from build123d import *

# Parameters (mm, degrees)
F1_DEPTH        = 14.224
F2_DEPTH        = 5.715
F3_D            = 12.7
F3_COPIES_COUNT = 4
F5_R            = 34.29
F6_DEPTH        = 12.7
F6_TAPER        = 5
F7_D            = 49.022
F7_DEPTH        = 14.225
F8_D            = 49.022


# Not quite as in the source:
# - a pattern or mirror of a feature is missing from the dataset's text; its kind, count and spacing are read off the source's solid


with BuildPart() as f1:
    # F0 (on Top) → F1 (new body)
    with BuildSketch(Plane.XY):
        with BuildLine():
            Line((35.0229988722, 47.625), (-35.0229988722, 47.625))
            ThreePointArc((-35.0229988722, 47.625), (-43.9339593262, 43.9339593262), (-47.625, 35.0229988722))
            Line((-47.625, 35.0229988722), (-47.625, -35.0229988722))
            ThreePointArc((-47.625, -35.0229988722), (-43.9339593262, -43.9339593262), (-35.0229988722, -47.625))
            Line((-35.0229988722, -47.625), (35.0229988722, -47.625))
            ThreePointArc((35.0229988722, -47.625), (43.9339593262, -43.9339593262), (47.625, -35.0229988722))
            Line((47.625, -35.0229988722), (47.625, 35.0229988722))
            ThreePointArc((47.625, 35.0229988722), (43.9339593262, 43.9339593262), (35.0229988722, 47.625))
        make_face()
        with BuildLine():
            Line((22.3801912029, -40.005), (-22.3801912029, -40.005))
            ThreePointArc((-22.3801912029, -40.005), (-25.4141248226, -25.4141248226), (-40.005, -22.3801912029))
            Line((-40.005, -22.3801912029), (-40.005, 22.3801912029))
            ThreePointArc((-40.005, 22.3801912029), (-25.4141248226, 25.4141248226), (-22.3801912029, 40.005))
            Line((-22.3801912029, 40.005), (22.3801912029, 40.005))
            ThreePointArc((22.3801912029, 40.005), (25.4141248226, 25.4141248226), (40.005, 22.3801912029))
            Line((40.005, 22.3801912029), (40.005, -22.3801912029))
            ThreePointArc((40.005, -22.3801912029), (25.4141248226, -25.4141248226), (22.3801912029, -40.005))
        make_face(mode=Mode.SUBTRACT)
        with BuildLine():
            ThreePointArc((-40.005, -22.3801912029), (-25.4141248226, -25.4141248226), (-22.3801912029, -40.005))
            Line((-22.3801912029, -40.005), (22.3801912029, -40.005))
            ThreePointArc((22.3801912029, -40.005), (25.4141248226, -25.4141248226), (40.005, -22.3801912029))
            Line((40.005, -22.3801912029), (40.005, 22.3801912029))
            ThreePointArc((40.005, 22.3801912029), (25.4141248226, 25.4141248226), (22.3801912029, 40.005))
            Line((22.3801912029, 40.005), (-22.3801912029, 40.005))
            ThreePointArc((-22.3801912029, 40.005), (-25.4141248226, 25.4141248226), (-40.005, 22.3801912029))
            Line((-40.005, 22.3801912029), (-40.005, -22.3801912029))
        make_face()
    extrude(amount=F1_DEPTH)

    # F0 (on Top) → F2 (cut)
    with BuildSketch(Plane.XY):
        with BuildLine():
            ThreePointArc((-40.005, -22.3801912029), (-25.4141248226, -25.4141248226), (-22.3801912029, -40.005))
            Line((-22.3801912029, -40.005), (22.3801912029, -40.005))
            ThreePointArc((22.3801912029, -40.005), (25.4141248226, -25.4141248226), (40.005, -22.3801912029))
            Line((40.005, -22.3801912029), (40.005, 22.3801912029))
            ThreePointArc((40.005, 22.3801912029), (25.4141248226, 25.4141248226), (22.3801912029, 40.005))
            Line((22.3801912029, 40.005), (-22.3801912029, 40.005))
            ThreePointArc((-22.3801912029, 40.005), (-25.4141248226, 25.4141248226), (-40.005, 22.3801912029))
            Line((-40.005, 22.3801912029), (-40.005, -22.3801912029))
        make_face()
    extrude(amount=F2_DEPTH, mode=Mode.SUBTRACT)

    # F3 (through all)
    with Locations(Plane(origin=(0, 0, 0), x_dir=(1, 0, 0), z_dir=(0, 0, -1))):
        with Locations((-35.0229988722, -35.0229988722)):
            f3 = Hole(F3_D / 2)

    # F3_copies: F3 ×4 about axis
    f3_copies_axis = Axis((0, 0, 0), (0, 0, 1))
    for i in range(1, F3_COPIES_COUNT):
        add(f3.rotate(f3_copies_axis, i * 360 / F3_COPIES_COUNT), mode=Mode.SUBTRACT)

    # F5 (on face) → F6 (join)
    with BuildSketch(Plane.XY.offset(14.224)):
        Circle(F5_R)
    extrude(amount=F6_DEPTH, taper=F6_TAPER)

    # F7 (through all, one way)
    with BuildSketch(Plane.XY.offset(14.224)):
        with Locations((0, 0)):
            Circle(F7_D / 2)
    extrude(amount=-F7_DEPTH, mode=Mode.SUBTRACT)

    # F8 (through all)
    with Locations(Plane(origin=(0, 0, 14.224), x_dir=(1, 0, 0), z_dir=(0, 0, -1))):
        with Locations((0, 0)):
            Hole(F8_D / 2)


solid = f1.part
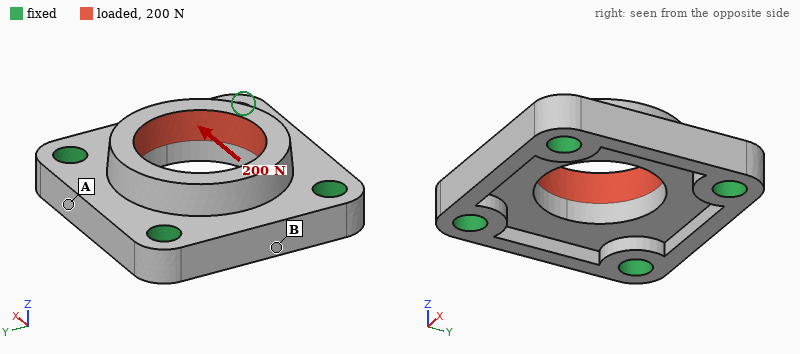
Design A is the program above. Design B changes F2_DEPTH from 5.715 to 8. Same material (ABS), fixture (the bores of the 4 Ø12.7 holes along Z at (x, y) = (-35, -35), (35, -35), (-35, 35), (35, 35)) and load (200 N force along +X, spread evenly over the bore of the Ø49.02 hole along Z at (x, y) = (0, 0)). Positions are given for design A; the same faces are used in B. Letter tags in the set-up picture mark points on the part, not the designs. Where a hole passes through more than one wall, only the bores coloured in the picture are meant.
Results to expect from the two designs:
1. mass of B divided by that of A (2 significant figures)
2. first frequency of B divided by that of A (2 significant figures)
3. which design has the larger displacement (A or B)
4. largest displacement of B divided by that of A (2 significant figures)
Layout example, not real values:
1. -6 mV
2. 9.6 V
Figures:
1. 0.92
2. 0.96
3. B
4. 1.1
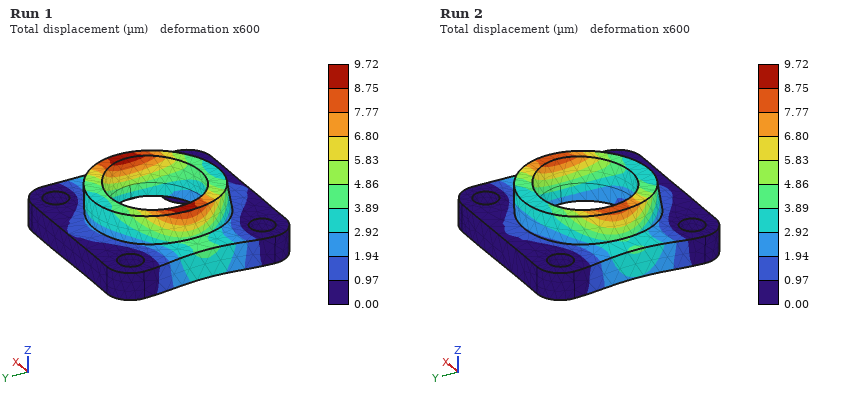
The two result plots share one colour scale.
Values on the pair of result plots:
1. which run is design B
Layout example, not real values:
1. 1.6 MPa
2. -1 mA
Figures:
1. Run 1
